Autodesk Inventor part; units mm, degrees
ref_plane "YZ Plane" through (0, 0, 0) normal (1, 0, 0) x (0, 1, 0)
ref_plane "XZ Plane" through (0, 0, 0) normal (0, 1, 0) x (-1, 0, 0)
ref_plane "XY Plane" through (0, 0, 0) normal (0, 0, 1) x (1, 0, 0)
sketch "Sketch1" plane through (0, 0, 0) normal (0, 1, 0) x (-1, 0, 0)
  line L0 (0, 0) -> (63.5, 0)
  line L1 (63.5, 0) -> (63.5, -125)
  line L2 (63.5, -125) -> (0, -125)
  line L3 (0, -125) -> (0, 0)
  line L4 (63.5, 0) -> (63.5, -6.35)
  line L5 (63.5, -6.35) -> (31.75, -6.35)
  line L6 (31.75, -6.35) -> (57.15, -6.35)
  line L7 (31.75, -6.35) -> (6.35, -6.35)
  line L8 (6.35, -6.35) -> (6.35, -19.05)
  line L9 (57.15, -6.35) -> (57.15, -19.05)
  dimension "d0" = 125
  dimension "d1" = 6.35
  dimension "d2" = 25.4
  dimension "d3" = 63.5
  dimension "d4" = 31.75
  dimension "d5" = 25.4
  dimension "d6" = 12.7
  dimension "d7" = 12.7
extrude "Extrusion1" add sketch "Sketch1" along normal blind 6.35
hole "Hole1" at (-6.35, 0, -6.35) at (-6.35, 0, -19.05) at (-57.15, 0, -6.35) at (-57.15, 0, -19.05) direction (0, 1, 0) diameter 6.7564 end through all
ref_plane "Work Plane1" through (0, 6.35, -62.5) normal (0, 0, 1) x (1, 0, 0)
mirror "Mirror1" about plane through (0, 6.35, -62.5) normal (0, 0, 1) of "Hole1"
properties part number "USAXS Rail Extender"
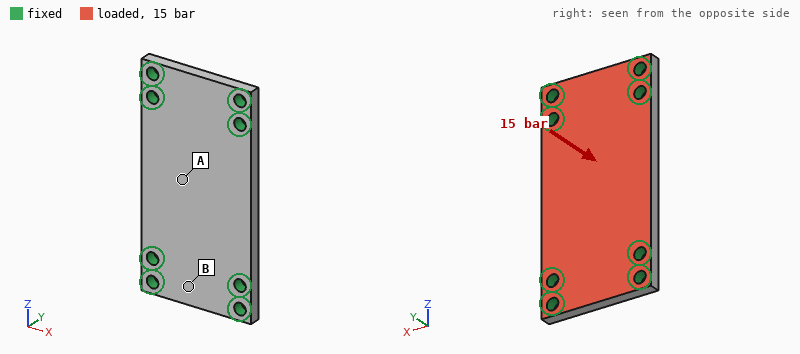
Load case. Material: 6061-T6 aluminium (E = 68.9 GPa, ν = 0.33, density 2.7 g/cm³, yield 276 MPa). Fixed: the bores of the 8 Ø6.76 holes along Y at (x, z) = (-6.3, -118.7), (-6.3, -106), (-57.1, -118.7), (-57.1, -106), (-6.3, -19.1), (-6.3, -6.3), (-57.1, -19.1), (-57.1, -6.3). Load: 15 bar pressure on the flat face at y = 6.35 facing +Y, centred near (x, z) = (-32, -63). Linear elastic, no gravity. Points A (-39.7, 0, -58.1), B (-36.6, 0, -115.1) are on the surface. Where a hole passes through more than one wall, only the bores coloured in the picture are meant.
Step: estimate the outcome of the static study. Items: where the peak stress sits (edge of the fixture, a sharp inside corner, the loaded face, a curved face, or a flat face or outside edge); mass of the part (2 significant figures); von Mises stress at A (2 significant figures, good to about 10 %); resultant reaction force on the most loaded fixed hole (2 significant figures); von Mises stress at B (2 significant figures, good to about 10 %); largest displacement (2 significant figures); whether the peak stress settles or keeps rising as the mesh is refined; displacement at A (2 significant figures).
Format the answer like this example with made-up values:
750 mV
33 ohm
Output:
edge of the fixture
130 g
61 MPa
2.8 kN
25 MPa
0.18 mm
keeps rising
0.17 mm
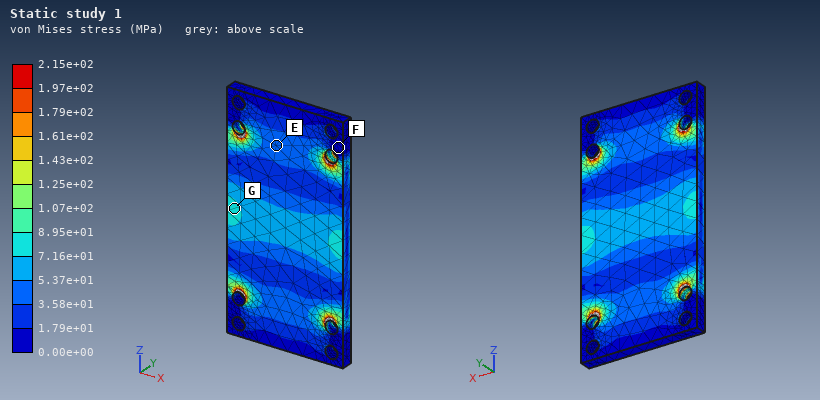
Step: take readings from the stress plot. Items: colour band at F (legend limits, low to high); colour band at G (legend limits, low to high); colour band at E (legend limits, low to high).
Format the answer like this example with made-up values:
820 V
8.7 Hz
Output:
0.00e+00 to 1.79e+01 MPa
7.16e+01 to 8.95e+01 MPa
3.58e+01 to 5.37e+01 MPa
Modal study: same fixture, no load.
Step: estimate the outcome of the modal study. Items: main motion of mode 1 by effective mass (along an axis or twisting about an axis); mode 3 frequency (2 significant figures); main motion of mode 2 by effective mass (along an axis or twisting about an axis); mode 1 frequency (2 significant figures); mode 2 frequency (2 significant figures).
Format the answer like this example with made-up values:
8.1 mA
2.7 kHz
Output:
along Y
10 kHz
twisting about Z
4100 Hz
6000 Hz
